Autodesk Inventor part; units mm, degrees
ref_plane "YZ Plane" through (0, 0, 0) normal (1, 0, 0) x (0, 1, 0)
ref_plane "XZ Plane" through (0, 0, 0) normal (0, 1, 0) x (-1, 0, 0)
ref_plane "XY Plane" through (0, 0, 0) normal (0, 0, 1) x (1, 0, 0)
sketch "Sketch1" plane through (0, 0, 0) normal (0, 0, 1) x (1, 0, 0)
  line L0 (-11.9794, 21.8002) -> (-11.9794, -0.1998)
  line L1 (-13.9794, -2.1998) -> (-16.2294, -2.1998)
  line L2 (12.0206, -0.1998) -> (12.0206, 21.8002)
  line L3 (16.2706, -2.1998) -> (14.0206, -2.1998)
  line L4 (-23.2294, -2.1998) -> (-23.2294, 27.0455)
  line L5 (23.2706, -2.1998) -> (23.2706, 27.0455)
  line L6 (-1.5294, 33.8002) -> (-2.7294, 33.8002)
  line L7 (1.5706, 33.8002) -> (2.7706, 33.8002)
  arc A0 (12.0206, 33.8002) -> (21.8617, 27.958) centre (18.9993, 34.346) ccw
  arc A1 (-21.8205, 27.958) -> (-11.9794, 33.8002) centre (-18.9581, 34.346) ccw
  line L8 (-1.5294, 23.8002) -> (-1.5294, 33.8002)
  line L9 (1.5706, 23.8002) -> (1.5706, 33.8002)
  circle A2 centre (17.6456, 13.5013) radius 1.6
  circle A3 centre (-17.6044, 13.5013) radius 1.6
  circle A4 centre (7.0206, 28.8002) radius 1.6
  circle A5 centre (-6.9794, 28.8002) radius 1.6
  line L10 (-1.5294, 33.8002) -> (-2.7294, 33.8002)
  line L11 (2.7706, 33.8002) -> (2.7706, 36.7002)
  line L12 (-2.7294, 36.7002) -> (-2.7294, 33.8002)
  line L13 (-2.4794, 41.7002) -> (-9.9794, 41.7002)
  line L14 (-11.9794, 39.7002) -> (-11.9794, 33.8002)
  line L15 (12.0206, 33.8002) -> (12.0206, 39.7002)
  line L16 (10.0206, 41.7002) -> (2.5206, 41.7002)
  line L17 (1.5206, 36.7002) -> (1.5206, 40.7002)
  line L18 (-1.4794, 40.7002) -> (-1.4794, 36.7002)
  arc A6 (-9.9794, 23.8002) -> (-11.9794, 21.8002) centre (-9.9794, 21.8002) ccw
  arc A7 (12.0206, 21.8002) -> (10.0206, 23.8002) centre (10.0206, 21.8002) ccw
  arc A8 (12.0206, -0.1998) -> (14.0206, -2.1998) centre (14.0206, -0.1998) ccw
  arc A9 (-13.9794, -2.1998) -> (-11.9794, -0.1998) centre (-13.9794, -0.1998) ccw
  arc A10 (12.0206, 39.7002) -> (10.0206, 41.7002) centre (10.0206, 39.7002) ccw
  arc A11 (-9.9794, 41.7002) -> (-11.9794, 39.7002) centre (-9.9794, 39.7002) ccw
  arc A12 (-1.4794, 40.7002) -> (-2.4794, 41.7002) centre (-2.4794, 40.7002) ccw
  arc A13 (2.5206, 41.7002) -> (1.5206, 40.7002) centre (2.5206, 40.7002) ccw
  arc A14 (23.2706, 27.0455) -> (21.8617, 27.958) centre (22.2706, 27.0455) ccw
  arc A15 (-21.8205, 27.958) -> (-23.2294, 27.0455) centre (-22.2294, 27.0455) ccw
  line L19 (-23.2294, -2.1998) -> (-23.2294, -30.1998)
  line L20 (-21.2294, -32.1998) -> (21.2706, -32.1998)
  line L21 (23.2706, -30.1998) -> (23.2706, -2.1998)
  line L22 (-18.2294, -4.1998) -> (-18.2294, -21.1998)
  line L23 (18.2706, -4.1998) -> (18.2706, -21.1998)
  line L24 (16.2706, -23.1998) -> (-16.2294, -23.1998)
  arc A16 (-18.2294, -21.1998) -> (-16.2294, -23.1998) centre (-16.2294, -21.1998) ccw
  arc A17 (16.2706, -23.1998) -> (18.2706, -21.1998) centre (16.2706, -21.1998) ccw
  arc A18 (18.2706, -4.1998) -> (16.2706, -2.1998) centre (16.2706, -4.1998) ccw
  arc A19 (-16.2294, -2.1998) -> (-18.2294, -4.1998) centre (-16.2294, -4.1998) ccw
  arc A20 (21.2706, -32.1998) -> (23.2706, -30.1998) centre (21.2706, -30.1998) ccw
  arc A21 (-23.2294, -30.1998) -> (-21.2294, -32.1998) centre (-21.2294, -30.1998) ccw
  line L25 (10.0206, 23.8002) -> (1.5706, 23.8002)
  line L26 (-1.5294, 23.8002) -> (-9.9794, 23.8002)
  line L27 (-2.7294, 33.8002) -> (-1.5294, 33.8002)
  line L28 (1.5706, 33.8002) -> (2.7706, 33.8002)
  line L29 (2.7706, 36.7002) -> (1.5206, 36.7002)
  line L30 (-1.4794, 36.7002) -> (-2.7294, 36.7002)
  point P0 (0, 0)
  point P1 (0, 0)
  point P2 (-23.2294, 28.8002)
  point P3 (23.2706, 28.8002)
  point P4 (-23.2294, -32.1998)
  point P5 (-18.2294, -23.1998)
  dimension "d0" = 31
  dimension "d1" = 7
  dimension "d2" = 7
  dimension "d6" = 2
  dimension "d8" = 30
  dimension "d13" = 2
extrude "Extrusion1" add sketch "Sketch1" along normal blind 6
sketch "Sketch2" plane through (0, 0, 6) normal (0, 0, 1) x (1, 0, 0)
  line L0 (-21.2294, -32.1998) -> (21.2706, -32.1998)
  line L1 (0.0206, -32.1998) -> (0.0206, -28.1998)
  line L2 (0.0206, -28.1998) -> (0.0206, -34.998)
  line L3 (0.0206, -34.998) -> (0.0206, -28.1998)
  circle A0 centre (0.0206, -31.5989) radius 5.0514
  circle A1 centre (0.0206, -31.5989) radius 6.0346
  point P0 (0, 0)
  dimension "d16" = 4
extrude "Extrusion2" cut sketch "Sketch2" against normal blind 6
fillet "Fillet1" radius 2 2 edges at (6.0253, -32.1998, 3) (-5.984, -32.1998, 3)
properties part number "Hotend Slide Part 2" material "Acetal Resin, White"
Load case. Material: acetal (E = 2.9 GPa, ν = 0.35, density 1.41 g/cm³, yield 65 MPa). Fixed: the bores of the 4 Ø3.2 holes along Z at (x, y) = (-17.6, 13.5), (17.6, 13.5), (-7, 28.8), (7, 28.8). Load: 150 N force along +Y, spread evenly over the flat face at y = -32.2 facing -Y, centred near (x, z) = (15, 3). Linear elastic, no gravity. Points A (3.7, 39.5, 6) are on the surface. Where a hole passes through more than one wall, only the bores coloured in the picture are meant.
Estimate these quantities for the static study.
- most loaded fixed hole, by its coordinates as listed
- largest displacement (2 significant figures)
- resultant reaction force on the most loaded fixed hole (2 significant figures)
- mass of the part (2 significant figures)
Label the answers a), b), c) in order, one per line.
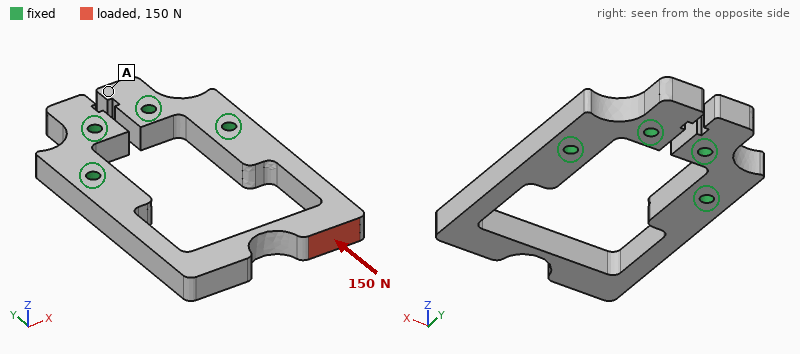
a) (17.6, 13.5)
b) 0.37 mm
c) 130 N
d) 13 g
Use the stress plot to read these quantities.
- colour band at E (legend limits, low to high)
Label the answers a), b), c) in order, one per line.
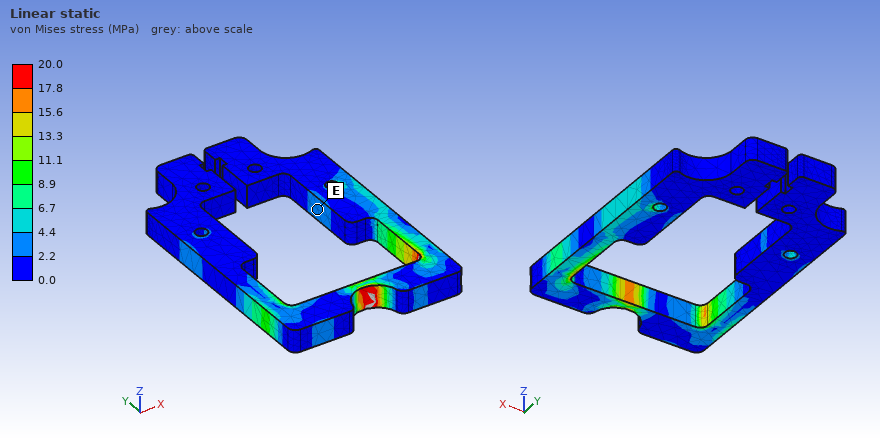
a) 2.2 to 4.4 MPa
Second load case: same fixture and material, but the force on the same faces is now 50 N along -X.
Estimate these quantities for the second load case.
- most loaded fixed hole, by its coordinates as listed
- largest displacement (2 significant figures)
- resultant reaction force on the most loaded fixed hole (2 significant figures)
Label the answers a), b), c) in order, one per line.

a) (-17.6, 13.5)
b) 0.45 mm
c) 69 N
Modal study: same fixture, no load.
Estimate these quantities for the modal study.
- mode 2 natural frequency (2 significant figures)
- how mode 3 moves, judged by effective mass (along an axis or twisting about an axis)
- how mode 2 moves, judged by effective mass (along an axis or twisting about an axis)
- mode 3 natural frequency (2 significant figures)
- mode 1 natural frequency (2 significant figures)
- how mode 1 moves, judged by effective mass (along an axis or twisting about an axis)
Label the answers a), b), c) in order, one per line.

a) 900 Hz
b) along X
c) twisting about Y
d) 990 Hz
e) 500 Hz
f) along Z
